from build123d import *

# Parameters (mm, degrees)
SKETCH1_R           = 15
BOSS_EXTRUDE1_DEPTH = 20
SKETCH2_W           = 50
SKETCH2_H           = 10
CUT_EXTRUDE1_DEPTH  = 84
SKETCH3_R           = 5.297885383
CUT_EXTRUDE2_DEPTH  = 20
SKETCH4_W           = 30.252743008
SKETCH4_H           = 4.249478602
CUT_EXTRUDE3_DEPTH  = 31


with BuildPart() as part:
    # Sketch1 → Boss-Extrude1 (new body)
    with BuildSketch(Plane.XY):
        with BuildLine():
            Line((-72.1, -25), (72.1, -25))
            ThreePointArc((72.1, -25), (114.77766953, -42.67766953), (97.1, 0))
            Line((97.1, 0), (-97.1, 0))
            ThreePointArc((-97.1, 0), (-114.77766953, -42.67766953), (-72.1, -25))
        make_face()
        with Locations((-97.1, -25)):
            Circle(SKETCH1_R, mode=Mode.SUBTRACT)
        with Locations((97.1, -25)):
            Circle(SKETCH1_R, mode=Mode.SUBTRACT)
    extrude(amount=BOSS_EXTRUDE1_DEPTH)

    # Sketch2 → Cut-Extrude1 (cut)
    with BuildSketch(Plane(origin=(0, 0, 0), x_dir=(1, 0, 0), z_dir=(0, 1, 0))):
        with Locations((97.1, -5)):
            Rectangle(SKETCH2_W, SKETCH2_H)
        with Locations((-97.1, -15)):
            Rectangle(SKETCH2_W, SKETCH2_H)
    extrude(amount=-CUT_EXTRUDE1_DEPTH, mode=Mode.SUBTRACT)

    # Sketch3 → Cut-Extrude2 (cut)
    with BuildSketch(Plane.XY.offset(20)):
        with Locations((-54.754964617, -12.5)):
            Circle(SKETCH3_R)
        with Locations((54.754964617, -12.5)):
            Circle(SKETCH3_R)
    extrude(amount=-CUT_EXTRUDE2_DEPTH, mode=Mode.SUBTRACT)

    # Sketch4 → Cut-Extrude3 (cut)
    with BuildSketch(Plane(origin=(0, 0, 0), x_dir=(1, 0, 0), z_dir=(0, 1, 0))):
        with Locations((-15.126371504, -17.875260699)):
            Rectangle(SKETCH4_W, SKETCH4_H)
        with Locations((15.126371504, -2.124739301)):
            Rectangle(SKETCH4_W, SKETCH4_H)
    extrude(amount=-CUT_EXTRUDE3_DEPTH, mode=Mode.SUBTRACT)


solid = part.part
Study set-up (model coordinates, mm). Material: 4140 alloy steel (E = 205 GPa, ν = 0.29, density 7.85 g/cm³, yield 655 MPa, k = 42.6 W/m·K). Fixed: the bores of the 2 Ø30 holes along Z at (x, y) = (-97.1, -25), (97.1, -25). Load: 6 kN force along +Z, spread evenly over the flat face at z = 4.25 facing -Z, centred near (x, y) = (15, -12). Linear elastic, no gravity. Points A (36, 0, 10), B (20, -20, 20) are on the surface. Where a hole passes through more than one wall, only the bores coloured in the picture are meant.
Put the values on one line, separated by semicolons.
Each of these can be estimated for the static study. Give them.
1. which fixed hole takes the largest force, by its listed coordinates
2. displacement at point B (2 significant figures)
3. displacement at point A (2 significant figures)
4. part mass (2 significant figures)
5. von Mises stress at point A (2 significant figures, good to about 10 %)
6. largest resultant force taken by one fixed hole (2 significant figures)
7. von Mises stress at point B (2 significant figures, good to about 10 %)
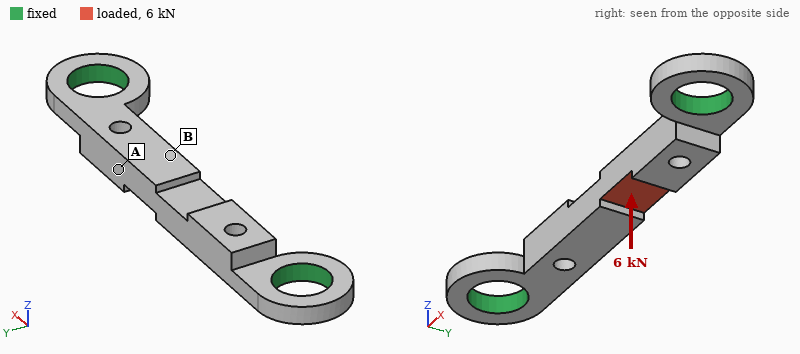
(97.1, -25); 0.15 mm; 0.13 mm; 710 g; 39 MPa; 3.7 kN; 120 MPa
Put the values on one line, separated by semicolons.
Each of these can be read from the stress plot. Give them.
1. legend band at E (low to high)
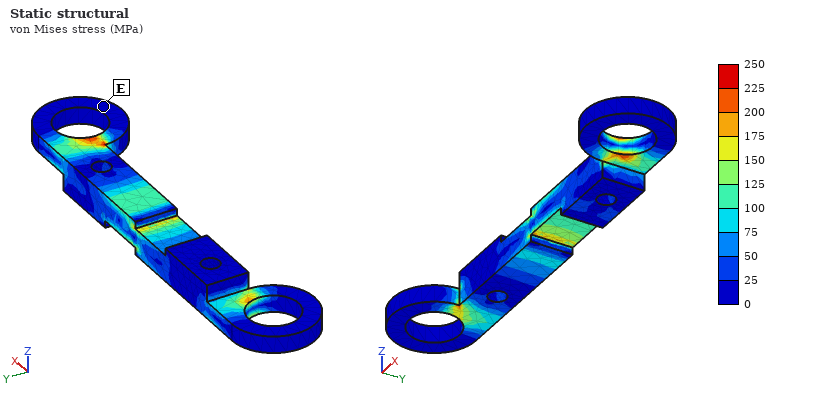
0 to 25 MPa
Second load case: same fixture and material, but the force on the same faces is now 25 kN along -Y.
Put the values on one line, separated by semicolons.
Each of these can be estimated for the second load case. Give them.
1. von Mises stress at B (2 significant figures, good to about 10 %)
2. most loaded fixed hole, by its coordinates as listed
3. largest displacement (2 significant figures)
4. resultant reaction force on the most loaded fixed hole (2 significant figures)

140 MPa; (97.1, -25); 0.25 mm; 17 kN
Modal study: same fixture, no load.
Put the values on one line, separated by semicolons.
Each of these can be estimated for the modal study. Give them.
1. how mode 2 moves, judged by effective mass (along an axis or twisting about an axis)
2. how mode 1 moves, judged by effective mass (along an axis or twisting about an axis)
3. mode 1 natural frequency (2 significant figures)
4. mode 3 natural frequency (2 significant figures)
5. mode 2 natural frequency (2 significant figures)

along Y; along Z; 1900 Hz; 6100 Hz; 3500 Hz
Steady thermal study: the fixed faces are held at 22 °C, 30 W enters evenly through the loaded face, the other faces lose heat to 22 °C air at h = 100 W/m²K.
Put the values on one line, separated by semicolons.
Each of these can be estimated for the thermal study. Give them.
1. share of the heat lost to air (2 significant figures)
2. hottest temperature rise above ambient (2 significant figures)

74 %; 39 K
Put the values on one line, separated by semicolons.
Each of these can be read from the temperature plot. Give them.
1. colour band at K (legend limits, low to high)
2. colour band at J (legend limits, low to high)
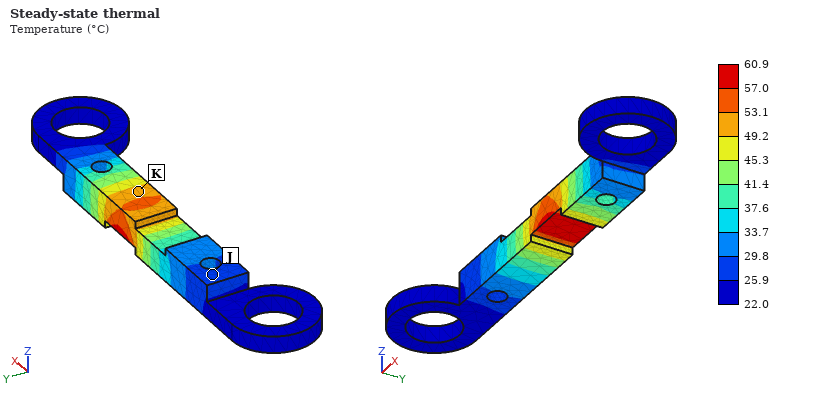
49.2 to 53.1 °C; 25.9 to 29.8 °C
